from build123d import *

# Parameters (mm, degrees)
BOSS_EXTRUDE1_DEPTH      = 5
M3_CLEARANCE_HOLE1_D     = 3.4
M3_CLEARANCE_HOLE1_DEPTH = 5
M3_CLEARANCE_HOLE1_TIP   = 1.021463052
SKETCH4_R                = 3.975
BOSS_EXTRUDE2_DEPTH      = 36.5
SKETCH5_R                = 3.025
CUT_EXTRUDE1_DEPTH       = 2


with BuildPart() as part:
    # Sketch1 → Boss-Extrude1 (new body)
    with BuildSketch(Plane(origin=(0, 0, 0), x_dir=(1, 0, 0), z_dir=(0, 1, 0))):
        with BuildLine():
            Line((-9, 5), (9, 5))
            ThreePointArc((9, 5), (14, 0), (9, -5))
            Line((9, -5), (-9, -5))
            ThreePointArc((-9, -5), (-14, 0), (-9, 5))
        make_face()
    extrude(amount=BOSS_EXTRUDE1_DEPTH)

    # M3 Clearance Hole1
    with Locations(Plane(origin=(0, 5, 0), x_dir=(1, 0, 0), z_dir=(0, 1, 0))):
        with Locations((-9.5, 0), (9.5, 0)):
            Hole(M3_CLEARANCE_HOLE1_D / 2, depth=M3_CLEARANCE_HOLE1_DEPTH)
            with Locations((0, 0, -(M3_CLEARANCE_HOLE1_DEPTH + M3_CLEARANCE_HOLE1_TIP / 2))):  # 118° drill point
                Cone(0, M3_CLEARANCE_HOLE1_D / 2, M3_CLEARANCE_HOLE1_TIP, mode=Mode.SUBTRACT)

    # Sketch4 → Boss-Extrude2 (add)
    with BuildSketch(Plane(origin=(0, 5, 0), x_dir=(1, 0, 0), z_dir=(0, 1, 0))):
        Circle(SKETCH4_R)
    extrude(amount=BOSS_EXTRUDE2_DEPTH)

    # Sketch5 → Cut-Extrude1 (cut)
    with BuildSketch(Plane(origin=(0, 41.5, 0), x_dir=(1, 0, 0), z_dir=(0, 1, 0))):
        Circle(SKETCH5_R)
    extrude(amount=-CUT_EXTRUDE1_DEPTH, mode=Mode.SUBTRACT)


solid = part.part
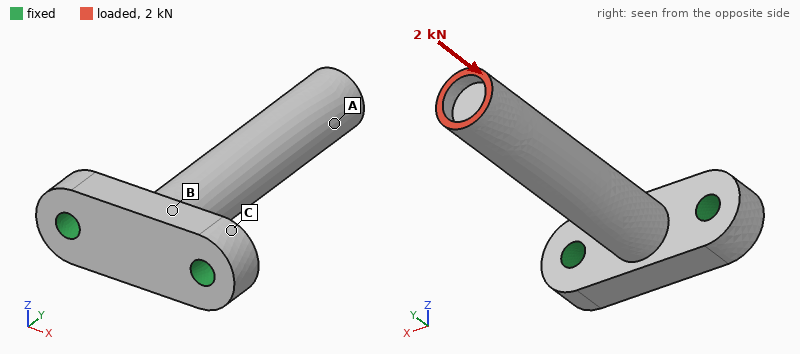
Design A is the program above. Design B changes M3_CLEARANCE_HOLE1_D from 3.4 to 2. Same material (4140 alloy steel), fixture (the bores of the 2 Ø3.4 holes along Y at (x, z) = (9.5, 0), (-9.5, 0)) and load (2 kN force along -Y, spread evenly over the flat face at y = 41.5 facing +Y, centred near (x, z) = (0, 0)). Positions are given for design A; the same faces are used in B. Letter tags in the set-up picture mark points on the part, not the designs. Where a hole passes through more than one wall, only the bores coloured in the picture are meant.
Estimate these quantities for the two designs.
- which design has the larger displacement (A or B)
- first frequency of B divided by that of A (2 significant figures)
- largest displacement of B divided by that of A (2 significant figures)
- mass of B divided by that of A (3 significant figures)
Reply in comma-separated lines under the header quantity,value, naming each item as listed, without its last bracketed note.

quantity,value
which design has the larger displacement,B
first frequency of B divided by that of A,0.96
largest displacement of B divided by that of A,1.1
mass of B divided by that of A,1.02
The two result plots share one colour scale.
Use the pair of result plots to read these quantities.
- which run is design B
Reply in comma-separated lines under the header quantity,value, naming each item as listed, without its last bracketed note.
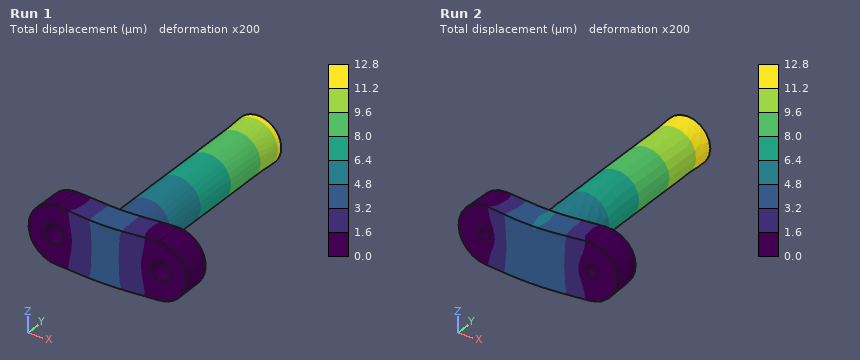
quantity,value
which run is design B,Run 2
